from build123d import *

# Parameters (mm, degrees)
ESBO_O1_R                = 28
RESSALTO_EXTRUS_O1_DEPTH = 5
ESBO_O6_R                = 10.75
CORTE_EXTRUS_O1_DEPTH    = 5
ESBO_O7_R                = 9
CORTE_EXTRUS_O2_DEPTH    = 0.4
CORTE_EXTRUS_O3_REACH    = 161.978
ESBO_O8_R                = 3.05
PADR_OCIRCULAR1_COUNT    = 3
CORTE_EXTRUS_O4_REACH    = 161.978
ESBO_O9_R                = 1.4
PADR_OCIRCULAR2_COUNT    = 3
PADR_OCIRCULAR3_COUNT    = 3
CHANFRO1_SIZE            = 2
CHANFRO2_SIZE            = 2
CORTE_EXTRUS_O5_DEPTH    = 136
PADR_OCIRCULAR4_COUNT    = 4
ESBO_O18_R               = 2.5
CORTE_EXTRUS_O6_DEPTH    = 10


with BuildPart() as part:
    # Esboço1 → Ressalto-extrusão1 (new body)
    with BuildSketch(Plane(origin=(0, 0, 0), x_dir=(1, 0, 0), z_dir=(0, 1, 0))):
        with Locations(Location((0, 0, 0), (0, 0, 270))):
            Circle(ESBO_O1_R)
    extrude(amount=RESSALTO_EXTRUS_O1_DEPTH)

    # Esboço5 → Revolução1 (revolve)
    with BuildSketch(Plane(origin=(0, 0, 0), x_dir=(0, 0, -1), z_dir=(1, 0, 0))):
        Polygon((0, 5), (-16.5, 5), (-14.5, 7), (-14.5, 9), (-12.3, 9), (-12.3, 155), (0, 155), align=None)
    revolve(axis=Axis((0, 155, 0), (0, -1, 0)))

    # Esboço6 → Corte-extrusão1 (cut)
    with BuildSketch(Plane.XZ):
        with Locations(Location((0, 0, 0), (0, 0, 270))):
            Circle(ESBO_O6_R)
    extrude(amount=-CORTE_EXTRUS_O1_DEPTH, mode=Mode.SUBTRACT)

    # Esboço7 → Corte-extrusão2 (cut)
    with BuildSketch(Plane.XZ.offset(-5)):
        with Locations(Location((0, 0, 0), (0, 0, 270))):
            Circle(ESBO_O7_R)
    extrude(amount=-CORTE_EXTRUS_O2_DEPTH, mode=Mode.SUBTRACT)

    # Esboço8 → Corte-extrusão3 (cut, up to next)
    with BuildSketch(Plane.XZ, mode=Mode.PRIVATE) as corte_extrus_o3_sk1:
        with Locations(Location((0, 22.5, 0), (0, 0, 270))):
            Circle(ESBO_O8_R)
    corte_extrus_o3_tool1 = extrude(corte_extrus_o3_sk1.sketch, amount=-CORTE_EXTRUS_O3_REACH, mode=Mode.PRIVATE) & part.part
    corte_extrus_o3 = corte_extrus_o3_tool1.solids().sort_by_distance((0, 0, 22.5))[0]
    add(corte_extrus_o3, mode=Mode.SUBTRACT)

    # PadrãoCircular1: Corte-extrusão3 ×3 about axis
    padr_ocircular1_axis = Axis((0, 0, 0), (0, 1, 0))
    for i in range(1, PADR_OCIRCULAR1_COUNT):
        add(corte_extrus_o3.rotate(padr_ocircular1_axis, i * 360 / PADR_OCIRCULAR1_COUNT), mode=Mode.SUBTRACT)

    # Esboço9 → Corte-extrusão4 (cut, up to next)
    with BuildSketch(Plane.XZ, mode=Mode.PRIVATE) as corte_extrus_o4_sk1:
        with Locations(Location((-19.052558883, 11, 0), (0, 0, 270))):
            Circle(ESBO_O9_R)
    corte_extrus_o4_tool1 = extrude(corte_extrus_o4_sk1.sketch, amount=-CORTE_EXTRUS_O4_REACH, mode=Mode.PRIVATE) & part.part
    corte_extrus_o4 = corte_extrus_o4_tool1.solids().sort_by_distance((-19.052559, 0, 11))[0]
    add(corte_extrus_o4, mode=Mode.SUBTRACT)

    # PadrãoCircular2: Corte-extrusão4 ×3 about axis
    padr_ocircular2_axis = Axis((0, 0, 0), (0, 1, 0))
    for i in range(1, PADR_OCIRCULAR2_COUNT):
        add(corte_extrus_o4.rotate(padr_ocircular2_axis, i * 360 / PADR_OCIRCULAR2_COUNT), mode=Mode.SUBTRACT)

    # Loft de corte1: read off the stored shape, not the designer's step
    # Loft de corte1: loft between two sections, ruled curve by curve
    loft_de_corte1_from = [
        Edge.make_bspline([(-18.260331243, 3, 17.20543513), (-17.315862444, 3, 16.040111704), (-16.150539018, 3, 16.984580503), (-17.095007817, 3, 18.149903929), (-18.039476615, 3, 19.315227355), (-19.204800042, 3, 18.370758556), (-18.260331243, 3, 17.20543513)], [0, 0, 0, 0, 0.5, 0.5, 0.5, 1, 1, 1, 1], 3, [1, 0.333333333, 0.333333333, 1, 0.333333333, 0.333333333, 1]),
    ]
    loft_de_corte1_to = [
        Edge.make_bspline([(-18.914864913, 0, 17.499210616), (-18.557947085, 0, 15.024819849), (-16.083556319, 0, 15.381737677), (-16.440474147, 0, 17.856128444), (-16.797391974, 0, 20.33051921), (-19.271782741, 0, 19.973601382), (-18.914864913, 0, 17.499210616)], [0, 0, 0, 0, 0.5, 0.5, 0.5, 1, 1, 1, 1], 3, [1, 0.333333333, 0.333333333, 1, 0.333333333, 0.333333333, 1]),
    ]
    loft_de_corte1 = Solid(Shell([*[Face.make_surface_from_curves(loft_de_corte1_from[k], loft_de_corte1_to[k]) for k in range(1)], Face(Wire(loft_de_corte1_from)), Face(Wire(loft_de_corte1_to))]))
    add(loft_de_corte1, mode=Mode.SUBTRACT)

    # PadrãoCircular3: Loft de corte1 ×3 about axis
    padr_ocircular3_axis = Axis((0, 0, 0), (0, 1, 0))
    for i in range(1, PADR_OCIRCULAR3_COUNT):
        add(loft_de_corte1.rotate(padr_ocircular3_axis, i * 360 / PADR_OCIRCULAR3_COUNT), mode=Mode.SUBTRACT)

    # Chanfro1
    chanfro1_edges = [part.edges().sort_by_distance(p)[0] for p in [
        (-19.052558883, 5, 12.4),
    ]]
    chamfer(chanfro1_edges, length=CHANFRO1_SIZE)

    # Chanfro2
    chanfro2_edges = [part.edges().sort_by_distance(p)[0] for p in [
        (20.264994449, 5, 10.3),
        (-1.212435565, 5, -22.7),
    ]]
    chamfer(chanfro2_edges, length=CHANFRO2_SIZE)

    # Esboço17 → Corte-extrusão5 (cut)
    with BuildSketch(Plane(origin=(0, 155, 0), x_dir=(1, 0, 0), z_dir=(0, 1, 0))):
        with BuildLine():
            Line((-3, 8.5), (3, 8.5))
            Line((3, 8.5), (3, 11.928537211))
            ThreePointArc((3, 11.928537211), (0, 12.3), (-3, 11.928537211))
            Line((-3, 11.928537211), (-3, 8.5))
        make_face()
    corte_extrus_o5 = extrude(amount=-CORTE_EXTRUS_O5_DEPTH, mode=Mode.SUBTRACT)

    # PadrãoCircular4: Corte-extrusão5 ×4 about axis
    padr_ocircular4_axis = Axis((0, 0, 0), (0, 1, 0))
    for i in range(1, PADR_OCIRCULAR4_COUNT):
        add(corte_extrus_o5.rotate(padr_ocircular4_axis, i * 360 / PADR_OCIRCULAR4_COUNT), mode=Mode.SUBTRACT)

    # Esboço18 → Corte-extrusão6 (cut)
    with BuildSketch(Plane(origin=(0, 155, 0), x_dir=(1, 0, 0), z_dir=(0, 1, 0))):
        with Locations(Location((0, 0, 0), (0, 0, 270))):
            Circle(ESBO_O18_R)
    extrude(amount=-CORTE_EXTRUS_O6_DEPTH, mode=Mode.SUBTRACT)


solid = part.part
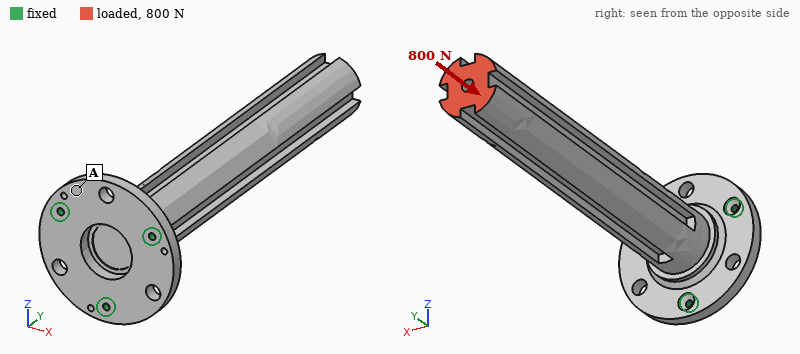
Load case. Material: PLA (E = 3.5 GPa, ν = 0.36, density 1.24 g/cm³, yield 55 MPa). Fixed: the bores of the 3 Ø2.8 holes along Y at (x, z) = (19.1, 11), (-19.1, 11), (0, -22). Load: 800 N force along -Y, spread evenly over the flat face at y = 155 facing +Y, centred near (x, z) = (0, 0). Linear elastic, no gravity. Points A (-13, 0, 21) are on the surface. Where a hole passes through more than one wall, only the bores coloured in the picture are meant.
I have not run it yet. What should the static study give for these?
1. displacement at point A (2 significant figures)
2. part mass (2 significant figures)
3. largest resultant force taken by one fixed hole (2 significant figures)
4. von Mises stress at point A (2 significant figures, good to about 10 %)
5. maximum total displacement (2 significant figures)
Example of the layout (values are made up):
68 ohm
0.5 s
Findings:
0.046 mm
87 g
360 N
2.7 MPa
0.17 mm
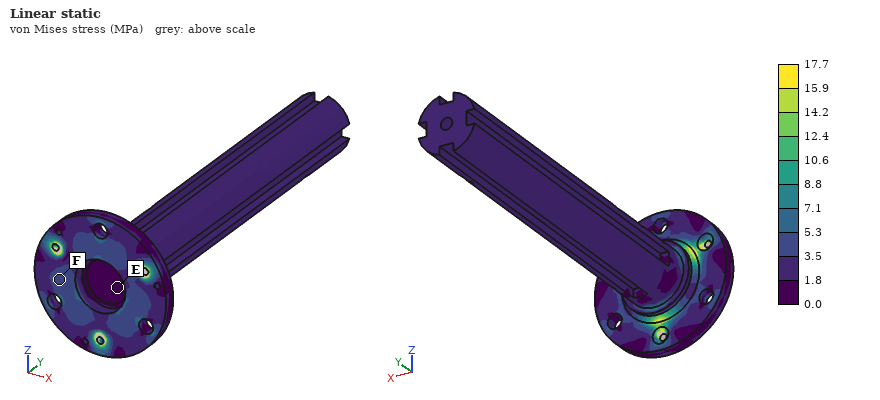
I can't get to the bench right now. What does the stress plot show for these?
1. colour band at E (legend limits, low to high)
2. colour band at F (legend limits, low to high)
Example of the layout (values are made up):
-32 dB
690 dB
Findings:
0.0 to 1.8 MPa
3.5 to 5.3 MPa
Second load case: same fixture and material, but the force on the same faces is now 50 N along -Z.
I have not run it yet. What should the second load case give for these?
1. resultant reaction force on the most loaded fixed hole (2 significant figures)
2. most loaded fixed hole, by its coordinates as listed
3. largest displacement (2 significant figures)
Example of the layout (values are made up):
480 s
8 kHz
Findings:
280 N
(0, -22)
1.9 mm
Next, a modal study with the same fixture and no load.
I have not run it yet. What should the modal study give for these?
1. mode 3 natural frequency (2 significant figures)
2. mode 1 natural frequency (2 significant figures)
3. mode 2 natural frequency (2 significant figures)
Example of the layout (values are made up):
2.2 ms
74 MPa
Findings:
1200 Hz
180 Hz
180 Hz
